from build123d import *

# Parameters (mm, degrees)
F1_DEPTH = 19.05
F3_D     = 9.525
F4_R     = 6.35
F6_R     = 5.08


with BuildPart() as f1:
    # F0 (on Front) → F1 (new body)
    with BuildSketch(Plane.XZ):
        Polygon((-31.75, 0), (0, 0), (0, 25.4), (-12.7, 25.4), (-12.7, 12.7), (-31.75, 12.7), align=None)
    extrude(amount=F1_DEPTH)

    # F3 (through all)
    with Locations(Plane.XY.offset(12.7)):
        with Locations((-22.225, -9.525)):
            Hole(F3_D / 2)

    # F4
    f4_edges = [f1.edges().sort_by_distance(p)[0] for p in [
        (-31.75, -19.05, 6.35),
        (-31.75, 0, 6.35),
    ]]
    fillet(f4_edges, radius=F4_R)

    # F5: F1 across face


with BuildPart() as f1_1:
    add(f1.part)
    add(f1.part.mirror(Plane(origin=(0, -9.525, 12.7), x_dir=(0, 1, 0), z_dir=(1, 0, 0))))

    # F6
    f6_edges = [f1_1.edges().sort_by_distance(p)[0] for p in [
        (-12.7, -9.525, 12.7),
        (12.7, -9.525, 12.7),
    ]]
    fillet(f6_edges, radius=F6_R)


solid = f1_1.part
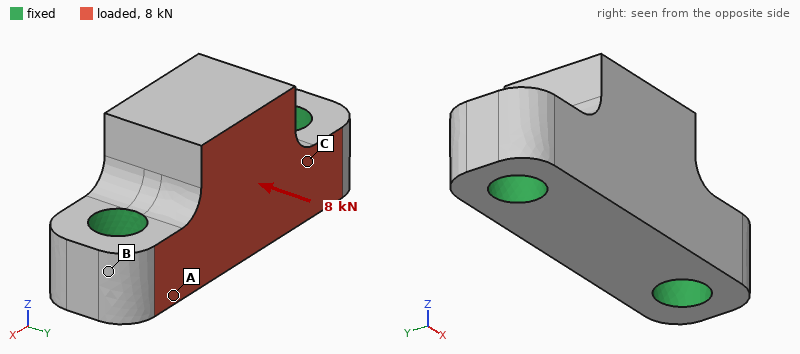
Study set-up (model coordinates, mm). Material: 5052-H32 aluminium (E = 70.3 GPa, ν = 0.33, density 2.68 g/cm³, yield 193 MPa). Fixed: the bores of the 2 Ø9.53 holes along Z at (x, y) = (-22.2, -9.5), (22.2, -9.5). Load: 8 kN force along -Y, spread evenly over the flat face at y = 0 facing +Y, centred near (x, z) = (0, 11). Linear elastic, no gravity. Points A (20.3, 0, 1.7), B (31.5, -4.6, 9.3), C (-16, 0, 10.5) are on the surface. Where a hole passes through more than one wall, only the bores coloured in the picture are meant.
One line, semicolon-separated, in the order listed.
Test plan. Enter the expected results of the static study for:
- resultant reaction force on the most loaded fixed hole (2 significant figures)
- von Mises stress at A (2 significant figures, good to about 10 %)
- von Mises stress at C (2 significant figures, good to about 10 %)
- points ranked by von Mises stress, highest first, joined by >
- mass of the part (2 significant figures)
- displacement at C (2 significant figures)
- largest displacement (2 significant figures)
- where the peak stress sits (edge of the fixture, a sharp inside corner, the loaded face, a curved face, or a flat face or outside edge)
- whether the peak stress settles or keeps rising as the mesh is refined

4.0 kN; 19 MPa; 37 MPa; C > A > B; 52 g; 6.6 µm; 24 µm; edge of the fixture; keeps rising
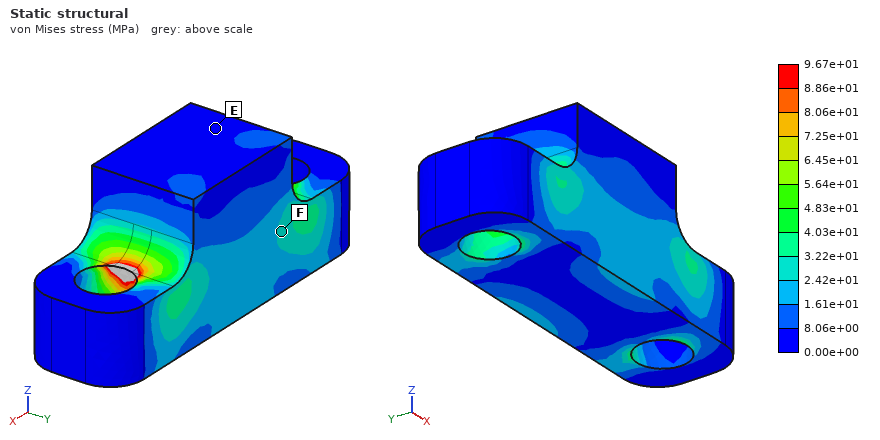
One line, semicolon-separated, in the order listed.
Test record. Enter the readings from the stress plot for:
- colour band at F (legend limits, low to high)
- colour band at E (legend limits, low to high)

2.42e+01 to 3.22e+01 MPa; 0.00e+00 to 8.06e+00 MPa
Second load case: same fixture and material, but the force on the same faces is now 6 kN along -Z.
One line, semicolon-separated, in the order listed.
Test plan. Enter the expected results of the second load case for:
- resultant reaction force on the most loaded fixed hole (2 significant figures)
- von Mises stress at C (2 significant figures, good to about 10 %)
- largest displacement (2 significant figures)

3.1 kN; 52 MPa; 25 µm
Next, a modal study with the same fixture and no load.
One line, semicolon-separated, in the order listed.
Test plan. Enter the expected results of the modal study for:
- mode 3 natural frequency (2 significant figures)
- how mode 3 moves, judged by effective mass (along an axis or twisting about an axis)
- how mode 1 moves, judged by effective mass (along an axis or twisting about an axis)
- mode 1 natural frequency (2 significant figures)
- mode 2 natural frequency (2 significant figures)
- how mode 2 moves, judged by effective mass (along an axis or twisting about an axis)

31 kHz; along Y; along Y; 15 kHz; 26 kHz; along Z
